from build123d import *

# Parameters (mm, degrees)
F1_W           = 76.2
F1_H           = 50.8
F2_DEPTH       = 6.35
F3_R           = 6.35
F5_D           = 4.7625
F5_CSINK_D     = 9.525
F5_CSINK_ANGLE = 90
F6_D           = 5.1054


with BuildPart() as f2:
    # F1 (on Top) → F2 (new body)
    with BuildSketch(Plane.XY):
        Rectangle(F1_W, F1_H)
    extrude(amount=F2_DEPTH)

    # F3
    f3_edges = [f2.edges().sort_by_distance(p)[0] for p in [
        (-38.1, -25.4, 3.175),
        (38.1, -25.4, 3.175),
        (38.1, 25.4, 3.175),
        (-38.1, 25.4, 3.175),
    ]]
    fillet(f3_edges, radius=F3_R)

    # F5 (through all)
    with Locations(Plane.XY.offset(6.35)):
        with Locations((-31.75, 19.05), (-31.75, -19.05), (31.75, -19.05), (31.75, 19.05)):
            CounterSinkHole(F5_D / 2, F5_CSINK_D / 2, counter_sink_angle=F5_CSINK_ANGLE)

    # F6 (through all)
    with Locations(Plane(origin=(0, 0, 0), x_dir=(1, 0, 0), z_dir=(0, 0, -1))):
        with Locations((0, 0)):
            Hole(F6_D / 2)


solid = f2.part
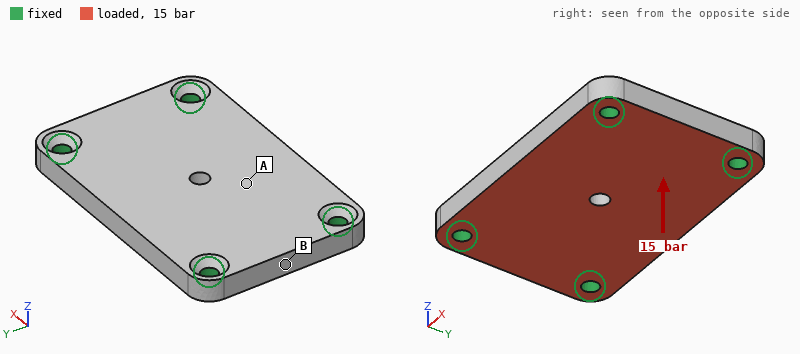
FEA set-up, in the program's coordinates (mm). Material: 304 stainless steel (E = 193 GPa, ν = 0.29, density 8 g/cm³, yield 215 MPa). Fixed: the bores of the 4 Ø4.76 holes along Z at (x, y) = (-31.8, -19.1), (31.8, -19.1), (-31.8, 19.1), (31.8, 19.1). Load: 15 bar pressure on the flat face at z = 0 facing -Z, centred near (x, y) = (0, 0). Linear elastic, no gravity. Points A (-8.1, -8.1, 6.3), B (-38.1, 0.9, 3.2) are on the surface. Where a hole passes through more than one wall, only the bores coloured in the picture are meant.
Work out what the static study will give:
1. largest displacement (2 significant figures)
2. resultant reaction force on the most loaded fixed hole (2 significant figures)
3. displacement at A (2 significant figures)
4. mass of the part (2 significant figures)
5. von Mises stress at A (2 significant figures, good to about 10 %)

29 µm
1.5 kN
25 µm
190 g
40 MPa
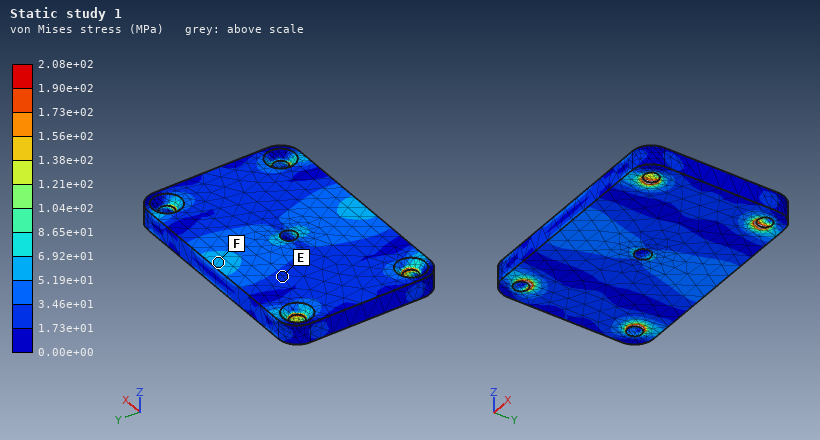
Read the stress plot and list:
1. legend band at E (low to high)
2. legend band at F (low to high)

1.73e+01 to 3.46e+01 MPa
5.19e+01 to 6.92e+01 MPa
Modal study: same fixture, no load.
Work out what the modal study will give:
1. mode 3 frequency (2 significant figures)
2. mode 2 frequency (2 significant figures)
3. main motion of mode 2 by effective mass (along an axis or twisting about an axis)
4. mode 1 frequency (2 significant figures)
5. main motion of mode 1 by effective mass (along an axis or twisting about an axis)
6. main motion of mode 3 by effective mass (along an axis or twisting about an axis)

15 kHz
8900 Hz
twisting about X
5900 Hz
along Z
twisting about Y
